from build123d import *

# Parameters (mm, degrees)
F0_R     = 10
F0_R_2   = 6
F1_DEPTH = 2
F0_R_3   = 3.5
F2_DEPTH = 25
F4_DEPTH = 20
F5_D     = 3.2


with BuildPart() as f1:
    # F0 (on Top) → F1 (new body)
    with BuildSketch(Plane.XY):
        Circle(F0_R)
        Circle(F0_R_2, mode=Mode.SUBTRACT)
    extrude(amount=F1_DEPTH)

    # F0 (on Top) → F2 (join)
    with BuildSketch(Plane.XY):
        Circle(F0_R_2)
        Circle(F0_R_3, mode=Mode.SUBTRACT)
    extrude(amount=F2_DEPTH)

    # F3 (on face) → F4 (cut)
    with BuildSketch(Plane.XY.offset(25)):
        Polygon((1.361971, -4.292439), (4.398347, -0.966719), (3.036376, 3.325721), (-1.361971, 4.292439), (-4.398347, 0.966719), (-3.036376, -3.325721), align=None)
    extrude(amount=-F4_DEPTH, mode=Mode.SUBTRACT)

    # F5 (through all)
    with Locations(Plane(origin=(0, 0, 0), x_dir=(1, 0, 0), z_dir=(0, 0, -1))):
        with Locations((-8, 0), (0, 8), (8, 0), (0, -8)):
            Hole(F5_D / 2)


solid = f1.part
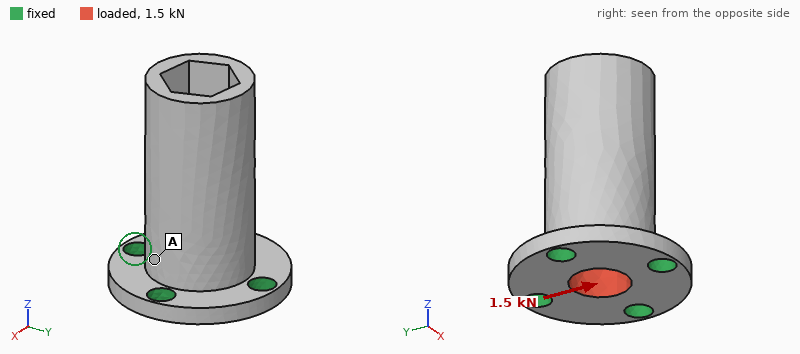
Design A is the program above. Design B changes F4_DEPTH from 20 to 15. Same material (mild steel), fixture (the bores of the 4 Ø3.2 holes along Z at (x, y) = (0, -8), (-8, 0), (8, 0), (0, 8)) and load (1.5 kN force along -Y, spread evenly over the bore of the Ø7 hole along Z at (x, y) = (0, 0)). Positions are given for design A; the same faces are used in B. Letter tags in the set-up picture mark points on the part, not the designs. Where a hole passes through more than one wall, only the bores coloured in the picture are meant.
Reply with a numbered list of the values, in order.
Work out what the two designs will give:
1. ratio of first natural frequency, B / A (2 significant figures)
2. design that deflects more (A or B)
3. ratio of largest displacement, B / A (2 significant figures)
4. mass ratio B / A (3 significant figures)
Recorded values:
1. 1.0
2. B
3. 4.1
4. 1.04
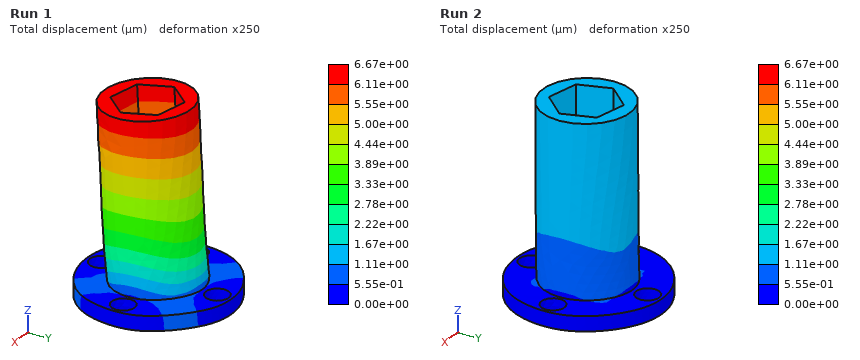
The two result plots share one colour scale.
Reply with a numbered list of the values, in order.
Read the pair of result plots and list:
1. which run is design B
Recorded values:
1. Run 1
